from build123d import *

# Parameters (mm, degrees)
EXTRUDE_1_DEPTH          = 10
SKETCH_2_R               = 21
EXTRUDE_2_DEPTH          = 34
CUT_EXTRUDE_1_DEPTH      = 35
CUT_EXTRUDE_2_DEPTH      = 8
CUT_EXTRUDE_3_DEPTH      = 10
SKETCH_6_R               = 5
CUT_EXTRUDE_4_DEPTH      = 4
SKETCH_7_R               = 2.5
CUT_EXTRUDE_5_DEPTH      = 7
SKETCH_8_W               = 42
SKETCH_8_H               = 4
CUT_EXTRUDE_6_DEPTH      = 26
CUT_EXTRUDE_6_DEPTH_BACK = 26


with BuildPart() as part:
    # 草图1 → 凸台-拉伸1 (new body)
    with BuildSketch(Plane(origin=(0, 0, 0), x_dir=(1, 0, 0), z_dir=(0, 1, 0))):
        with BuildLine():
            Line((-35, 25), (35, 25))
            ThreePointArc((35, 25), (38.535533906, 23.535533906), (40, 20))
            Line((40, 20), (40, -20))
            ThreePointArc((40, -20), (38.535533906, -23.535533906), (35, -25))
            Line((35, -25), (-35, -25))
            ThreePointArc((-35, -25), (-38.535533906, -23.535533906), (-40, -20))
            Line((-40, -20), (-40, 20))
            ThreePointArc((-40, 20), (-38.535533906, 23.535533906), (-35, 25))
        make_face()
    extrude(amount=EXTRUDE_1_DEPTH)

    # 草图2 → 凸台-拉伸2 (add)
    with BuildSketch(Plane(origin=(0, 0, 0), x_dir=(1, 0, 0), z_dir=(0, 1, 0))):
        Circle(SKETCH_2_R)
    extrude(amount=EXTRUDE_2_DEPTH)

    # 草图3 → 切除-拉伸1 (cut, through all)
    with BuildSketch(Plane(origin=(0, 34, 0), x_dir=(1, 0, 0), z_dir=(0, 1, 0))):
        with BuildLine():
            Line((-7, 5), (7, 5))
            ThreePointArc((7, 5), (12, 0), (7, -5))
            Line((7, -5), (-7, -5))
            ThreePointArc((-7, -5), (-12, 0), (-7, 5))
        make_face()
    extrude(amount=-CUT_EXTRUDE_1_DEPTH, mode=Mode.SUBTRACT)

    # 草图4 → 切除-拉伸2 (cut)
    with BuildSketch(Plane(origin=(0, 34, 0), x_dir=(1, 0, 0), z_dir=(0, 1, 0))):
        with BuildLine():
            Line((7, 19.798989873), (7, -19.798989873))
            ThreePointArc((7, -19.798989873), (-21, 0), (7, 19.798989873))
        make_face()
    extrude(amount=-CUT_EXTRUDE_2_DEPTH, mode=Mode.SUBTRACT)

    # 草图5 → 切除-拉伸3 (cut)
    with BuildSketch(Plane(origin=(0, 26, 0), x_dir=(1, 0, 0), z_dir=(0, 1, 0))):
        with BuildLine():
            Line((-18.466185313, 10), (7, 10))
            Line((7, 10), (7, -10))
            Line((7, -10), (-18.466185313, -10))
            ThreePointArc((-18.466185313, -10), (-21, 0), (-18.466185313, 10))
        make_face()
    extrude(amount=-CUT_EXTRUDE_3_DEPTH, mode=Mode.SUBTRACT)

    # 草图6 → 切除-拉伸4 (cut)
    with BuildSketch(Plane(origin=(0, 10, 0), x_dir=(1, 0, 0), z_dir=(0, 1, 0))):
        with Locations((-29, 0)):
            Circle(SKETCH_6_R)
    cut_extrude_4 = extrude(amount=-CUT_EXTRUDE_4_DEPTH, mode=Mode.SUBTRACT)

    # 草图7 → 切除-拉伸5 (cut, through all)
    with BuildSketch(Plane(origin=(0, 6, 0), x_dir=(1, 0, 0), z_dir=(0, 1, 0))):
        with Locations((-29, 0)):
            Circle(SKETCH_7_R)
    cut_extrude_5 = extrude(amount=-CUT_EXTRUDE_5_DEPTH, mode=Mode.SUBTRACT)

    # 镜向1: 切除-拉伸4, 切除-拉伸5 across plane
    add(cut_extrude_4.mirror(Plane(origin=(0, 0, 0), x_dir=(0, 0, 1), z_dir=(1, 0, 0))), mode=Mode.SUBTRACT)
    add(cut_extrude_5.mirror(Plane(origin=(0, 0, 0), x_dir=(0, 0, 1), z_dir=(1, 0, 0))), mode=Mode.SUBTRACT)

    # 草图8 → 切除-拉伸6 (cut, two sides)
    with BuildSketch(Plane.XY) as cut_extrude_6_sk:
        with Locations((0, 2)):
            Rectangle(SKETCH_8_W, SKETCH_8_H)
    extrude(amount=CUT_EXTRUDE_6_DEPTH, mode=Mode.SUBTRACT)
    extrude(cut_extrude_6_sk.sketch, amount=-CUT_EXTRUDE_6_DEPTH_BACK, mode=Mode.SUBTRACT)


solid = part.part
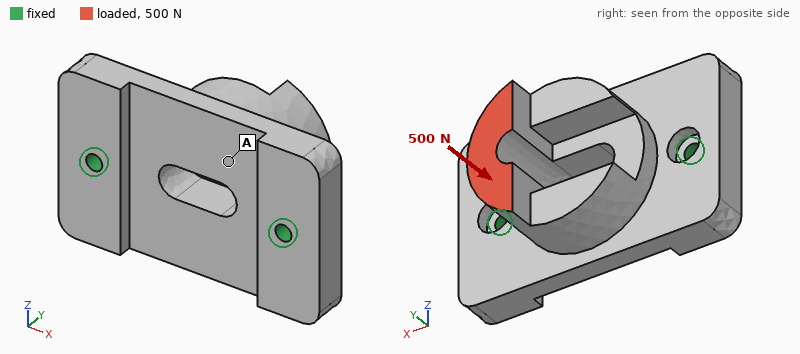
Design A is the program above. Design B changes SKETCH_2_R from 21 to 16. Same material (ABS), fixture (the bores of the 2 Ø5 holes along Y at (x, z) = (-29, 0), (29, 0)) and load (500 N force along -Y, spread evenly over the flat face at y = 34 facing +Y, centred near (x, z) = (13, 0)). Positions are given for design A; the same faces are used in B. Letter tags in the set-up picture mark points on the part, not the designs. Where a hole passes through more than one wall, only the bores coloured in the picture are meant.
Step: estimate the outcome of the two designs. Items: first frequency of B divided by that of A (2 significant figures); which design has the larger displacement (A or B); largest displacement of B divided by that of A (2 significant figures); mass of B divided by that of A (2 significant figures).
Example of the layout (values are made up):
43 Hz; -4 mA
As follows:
1.2; B; 2.2; 0.79
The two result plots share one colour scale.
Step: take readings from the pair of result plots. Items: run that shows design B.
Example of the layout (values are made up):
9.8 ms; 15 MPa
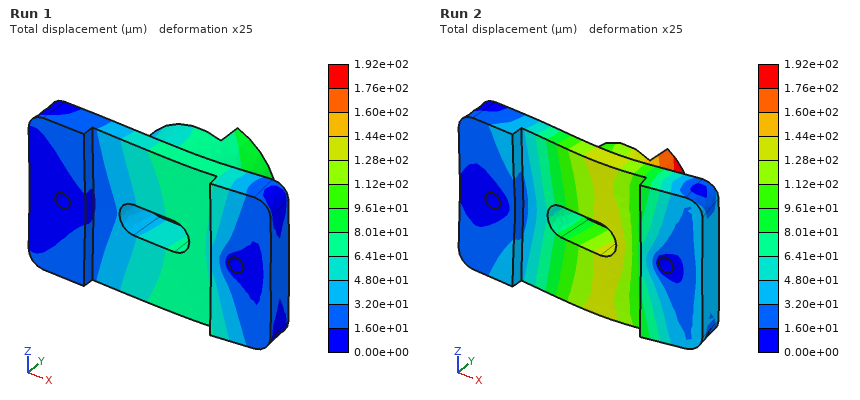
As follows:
Run 2
